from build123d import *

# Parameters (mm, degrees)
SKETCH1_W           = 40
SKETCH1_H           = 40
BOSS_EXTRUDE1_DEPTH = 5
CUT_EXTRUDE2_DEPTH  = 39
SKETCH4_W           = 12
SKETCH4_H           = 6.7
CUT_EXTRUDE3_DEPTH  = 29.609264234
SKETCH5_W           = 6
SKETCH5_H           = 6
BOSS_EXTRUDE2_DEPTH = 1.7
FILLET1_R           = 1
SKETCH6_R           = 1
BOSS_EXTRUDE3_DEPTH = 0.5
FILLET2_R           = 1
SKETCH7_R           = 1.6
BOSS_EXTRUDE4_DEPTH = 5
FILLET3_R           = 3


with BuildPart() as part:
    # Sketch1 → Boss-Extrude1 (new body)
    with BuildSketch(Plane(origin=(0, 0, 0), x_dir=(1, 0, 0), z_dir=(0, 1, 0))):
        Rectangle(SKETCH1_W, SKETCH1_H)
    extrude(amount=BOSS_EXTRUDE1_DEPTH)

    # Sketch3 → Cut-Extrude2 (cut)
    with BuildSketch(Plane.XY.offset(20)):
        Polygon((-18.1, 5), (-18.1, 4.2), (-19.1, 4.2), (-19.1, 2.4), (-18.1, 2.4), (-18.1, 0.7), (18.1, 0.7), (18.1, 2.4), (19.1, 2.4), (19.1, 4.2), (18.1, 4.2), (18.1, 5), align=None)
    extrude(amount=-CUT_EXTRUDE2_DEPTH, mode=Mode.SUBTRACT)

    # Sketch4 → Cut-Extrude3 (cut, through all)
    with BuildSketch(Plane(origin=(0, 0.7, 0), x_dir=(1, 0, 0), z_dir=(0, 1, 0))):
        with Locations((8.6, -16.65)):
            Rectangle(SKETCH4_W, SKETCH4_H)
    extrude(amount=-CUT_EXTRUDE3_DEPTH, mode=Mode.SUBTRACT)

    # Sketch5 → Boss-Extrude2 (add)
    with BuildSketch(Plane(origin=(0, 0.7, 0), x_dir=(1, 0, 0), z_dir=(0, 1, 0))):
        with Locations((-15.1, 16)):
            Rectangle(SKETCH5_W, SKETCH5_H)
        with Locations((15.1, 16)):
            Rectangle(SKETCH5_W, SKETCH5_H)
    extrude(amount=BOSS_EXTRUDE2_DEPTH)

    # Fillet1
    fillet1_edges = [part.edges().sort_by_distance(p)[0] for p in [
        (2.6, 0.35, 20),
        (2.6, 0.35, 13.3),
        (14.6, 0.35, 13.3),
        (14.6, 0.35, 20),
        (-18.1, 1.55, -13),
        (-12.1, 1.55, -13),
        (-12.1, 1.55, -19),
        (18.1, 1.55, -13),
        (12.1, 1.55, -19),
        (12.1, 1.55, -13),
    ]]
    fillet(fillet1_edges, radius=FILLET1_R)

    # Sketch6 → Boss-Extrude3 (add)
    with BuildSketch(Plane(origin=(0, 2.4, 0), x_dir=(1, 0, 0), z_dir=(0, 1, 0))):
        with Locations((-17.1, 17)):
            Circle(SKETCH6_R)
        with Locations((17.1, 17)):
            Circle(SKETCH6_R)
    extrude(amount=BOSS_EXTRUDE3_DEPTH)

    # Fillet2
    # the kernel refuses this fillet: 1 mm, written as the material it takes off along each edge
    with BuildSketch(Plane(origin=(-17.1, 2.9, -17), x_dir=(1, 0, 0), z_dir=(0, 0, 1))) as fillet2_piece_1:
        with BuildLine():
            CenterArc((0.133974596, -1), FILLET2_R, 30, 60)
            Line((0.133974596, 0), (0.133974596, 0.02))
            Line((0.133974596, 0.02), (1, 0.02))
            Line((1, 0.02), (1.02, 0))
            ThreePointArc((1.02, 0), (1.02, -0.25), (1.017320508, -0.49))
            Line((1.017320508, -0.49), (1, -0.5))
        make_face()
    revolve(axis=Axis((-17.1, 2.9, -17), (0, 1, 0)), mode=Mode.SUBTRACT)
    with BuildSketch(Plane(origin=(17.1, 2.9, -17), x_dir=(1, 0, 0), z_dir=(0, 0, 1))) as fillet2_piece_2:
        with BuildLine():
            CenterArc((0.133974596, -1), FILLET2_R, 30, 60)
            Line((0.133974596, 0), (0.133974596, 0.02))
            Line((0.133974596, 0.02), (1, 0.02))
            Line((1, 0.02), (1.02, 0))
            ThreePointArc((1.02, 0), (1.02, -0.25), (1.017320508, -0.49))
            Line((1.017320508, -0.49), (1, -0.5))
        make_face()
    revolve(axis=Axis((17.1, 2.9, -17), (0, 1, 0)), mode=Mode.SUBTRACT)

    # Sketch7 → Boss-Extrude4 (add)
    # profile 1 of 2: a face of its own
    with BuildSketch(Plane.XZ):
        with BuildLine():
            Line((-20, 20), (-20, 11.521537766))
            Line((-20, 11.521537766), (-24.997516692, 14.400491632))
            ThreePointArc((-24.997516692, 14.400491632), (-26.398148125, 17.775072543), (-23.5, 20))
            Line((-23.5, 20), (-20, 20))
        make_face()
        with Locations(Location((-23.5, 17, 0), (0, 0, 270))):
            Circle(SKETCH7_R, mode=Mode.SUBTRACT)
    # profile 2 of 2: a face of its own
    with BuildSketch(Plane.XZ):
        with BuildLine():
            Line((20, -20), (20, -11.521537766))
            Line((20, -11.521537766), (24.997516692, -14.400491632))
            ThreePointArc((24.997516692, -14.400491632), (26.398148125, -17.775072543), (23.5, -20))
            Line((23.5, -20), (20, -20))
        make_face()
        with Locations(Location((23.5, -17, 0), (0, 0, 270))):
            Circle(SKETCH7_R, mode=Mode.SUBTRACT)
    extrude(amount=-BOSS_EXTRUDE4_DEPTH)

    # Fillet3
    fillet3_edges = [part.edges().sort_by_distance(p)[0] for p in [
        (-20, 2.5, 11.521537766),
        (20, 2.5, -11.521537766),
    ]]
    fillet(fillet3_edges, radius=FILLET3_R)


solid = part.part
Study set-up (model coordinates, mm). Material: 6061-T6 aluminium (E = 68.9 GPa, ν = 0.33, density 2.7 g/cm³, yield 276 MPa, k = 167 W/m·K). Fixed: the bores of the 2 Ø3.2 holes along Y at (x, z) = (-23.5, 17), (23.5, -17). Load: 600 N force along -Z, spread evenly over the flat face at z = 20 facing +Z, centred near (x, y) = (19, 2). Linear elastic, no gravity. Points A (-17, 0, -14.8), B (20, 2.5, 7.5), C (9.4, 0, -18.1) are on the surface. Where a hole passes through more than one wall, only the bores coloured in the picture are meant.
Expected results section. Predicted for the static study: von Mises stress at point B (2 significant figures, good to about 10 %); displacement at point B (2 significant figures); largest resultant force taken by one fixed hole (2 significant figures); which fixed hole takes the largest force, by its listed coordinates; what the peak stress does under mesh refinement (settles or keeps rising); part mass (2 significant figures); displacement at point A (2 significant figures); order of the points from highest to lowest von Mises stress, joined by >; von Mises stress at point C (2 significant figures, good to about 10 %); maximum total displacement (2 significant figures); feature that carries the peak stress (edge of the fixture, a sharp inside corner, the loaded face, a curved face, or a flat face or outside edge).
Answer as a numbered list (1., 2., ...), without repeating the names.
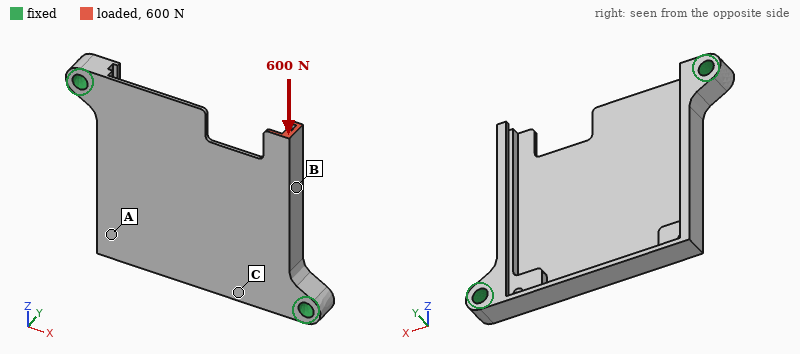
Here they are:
1. 68 MPa
2. 25 µm
3. 540 N
4. (23.5, -17)
5. keeps rising
6. 5.9 g
7. 27 µm
8. B > C > A
9. 20 MPa
10. 48 µm
11. edge of the fixture
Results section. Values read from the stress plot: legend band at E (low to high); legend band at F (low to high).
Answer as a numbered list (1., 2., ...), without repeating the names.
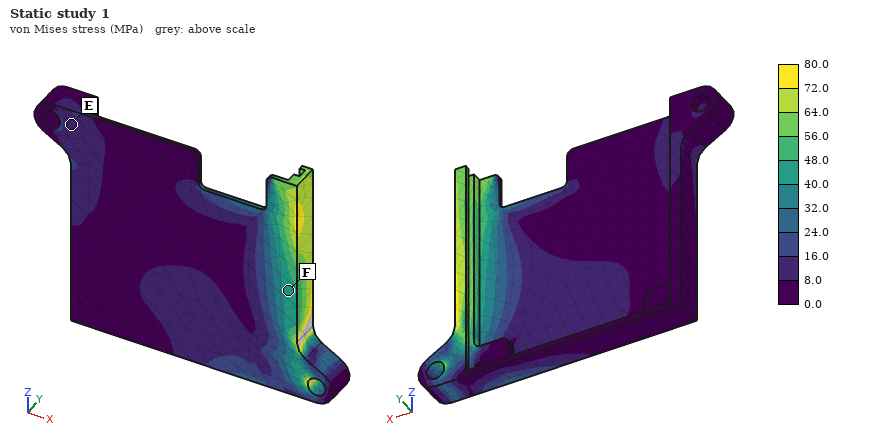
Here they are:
1. 8.0 to 16.0 MPa
2. 40.0 to 48.0 MPa
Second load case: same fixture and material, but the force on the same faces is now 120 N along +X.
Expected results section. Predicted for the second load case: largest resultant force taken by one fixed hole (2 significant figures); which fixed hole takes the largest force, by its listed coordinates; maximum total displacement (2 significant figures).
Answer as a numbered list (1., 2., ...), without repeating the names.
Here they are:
1. 90 N
2. (-23.5, 17)
3. 0.25 mm
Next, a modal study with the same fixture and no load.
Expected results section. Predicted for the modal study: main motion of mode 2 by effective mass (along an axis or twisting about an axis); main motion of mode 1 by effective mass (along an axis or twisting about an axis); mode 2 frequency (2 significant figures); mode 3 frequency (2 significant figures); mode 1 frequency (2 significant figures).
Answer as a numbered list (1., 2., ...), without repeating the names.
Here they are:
1. along Y
2. along Y
3. 3100 Hz
4. 3800 Hz
5. 2300 Hz
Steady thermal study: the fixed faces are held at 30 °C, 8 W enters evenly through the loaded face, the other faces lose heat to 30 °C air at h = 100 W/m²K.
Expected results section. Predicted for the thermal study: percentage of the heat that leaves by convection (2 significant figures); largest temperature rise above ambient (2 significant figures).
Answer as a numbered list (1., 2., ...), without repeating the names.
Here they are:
1. 55 %
2. 84 K
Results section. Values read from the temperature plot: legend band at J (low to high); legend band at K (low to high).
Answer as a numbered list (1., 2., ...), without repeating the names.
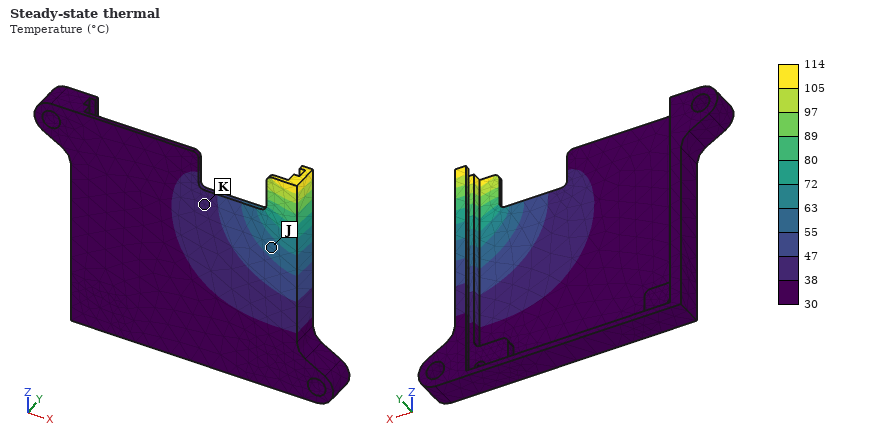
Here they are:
1. 55 to 63 °C
2. 38 to 47 °C
